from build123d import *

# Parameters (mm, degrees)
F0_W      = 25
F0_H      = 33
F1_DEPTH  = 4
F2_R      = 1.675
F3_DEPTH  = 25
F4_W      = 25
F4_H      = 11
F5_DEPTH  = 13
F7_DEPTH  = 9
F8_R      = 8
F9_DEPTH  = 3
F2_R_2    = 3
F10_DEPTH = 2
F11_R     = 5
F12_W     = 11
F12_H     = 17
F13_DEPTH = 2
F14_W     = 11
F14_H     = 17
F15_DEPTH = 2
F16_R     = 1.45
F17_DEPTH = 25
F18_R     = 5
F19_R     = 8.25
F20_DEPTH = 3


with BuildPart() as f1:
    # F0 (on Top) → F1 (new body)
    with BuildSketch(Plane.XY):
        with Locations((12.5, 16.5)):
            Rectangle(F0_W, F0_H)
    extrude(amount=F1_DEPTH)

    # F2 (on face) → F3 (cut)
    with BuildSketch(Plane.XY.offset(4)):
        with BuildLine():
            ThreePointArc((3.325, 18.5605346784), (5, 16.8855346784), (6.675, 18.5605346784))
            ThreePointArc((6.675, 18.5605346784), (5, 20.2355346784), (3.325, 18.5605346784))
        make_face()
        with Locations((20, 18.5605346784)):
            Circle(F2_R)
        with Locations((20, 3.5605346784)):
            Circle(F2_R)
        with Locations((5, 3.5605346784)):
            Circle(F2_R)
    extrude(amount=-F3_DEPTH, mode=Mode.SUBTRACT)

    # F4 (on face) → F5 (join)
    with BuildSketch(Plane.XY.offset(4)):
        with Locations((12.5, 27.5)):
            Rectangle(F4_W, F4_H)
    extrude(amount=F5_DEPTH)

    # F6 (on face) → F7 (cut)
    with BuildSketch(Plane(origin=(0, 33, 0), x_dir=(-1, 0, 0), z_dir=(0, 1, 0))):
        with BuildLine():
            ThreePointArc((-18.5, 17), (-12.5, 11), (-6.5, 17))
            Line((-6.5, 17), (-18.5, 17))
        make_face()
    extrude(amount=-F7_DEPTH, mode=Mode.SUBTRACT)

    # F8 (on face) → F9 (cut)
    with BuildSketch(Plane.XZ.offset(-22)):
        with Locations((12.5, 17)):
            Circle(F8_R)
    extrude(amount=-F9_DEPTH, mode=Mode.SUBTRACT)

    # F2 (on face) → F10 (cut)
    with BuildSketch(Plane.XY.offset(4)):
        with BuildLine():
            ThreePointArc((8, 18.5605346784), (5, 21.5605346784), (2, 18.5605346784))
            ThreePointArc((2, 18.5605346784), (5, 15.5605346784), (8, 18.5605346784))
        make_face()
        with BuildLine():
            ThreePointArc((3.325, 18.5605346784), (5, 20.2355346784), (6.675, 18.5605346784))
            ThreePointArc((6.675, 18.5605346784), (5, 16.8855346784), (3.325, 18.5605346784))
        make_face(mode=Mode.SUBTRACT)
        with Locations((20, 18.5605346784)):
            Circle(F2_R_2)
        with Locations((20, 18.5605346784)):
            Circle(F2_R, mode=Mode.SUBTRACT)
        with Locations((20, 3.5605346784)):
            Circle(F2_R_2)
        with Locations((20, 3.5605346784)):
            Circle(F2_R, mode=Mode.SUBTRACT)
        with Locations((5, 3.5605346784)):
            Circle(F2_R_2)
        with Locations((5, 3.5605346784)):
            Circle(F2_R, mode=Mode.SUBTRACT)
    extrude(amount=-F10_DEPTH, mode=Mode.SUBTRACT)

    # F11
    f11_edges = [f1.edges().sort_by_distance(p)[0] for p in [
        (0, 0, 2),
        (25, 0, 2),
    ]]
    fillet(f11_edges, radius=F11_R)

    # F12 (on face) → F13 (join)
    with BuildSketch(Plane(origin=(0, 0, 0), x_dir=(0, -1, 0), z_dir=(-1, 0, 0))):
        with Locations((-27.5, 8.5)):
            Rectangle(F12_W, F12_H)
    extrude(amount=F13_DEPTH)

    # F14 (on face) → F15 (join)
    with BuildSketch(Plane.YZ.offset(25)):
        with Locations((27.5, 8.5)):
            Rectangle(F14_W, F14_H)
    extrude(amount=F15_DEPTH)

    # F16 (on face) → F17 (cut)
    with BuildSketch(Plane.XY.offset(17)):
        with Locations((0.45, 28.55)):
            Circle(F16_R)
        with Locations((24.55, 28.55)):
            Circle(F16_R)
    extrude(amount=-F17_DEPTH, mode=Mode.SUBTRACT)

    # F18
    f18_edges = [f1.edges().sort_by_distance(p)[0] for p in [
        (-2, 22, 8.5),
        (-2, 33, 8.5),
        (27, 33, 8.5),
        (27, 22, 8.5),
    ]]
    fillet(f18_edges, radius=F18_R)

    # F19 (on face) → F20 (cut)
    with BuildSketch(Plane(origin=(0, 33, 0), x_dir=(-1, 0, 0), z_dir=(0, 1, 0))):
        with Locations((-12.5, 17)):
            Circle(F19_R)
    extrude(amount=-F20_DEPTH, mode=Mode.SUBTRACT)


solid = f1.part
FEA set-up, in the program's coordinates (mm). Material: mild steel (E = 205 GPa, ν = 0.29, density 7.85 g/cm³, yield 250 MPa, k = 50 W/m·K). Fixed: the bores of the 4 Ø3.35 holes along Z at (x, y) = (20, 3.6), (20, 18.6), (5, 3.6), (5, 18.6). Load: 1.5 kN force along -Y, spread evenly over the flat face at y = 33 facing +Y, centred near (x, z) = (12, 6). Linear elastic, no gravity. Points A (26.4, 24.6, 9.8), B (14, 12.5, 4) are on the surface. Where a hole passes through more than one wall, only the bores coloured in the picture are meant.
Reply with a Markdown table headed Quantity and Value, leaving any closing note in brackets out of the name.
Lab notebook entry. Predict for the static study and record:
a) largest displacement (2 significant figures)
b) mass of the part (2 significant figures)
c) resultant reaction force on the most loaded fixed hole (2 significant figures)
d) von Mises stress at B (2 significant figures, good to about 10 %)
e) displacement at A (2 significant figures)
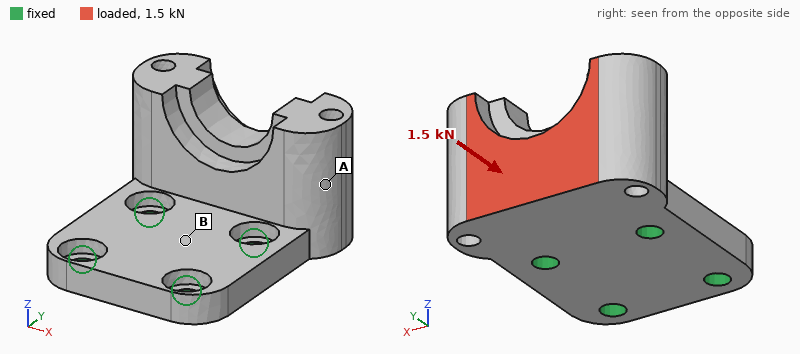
| Quantity | Value |
|---|---|
| largest displacement | 42 µm |
| mass of the part | 46 g |
| resultant reaction force on the most loaded fixed hole | 450 N |
| von Mises stress at B | 34 MPa |
| displacement at A | 19 µm |
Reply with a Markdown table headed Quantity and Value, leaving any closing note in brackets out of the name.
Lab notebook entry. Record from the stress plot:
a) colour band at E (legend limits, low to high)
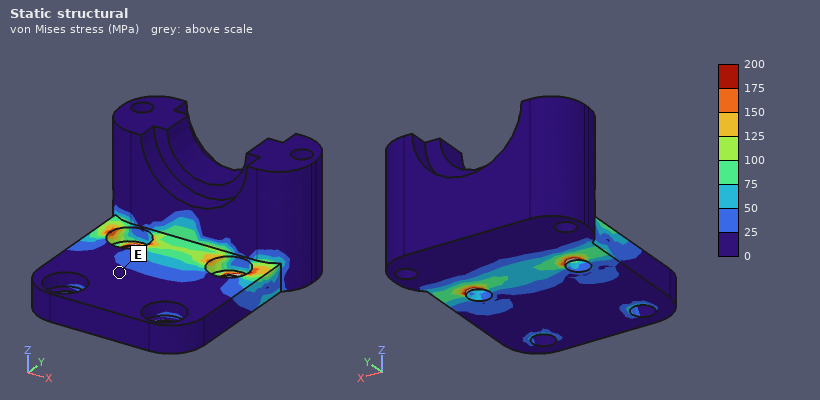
| Quantity | Value |
|---|---|
| colour band at E | 0 to 25 MPa |
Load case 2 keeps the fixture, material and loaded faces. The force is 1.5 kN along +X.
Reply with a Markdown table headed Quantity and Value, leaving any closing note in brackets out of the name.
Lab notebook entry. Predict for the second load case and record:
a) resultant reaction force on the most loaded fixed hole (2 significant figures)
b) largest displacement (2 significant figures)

| Quantity | Value |
|---|---|
| resultant reaction force on the most loaded fixed hole | 1.4 kN |
| largest displacement | 7.4 µm |
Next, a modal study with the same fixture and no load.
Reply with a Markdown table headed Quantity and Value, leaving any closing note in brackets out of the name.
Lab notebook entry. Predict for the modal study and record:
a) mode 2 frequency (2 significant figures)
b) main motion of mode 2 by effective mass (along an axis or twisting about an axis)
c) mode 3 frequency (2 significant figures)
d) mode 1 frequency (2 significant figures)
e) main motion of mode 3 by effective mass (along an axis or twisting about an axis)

| Quantity | Value |
|---|---|
| mode 2 frequency | 12 kHz |
| main motion of mode 2 by effective mass | along X |
| mode 3 frequency | 19 kHz |
| mode 1 frequency | 4900 Hz |
| main motion of mode 3 by effective mass | along X |
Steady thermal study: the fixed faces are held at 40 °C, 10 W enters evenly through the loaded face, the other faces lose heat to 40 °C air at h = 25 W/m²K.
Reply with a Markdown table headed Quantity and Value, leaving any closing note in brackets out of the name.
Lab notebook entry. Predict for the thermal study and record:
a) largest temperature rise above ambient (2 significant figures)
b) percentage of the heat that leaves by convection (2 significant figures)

| Quantity | Value |
|---|---|
| largest temperature rise above ambient | 22 K |
| percentage of the heat that leaves by convection | 8.5 % |
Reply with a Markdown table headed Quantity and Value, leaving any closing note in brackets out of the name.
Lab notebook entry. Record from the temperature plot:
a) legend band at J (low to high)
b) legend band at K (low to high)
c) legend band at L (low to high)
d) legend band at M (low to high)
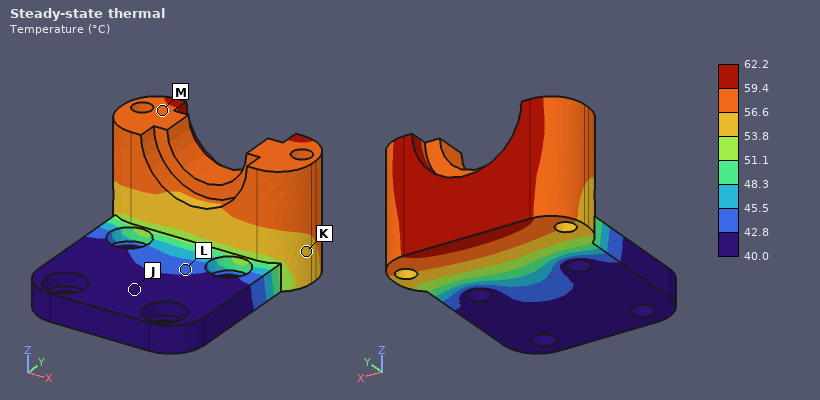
| Quantity | Value |
|---|---|
| legend band at J | 40.0 to 42.8 °C |
| legend band at K | 53.8 to 56.6 °C |
| legend band at L | 42.8 to 45.5 °C |
| legend band at M | 56.6 to 59.4 °C |
